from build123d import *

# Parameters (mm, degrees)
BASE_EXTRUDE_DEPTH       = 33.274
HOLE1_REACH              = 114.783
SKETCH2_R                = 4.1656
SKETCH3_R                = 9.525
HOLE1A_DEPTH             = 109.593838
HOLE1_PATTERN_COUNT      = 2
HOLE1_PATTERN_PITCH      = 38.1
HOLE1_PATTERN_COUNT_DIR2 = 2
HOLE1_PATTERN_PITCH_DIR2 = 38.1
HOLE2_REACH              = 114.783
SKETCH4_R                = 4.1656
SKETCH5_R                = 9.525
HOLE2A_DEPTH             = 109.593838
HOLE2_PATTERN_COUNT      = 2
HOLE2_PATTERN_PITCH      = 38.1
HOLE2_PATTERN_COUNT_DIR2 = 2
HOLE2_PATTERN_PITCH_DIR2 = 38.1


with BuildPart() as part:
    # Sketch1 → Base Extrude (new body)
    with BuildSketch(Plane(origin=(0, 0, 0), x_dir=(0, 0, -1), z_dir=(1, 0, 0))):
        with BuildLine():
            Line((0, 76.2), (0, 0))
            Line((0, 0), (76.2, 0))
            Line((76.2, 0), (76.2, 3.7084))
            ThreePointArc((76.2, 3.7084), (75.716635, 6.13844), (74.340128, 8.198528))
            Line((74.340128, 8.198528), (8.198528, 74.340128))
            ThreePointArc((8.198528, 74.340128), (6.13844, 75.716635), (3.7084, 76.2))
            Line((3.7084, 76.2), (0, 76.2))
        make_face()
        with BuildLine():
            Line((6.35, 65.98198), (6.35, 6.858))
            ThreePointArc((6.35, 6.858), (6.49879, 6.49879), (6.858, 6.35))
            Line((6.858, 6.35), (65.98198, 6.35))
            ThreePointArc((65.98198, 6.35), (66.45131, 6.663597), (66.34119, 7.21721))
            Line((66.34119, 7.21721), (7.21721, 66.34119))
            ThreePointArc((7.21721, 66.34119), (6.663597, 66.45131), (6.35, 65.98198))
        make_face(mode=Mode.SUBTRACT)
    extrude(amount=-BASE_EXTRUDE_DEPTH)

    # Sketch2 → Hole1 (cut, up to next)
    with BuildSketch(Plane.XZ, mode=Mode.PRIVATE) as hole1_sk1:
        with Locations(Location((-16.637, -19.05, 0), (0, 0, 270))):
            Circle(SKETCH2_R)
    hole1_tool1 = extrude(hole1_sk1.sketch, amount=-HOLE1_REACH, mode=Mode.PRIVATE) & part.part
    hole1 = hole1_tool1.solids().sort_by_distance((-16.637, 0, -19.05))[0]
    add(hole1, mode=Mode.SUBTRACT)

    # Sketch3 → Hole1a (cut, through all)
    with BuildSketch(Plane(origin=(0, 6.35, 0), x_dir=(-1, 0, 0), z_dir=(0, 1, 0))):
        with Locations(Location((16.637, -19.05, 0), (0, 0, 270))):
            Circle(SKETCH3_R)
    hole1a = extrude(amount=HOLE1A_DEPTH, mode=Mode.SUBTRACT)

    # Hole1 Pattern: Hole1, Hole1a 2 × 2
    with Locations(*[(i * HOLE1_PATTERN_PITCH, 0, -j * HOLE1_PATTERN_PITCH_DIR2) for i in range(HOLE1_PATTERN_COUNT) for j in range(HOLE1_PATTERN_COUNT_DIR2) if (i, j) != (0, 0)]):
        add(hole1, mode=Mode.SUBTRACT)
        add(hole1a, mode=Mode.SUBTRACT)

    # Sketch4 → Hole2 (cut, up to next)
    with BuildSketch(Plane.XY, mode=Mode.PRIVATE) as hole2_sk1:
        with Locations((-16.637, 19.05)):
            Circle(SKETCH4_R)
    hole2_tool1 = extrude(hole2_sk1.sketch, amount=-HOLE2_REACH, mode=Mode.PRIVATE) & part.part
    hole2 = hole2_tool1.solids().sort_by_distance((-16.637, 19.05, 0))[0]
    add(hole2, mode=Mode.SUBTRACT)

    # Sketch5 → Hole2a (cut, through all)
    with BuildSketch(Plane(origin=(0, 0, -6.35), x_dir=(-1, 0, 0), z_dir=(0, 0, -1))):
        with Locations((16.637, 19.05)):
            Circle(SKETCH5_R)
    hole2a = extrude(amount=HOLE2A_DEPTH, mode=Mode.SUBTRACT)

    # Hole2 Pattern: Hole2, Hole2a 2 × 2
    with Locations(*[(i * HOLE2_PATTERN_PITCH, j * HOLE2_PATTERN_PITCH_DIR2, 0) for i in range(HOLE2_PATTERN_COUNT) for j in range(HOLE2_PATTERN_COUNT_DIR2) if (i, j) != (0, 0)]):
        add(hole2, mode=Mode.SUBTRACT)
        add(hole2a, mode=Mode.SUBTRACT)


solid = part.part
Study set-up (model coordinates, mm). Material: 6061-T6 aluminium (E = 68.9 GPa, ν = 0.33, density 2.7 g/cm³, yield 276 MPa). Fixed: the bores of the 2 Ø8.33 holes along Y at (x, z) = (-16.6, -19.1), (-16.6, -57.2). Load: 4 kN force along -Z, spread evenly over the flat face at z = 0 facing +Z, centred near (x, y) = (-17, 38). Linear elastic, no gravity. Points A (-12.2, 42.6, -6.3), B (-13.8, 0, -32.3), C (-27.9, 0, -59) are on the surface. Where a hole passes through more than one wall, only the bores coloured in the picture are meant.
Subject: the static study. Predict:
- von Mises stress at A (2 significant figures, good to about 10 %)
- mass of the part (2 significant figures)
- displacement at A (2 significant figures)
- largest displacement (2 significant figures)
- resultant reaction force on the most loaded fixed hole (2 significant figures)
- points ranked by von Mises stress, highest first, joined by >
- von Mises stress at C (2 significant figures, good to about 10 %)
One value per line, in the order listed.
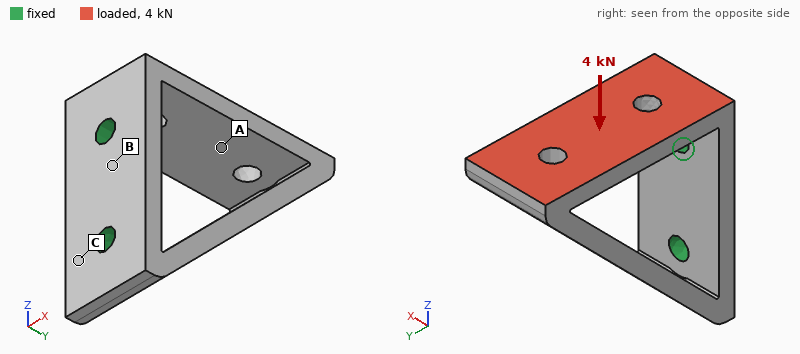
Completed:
88 MPa
120 g
0.31 mm
0.33 mm
2.9 kN
A > C > B
52 MPa
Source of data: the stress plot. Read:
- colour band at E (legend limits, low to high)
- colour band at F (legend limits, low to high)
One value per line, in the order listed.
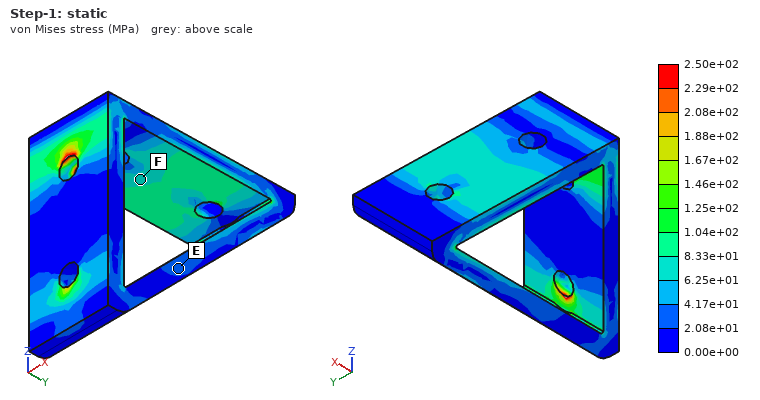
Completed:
2.08e+01 to 4.17e+01 MPa
6.25e+01 to 8.33e+01 MPa
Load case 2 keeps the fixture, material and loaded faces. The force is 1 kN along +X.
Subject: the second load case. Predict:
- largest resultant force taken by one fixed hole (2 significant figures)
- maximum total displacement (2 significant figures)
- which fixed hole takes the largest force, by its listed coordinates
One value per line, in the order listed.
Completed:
1.2 kN
0.24 mm
(-16.6, -19.1)
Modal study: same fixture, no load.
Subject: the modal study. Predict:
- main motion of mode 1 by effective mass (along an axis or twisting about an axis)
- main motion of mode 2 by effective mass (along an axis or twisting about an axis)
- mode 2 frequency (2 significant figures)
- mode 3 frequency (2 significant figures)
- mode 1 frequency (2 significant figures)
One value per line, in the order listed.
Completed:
along X
along Z
2000 Hz
3900 Hz
1400 Hz
